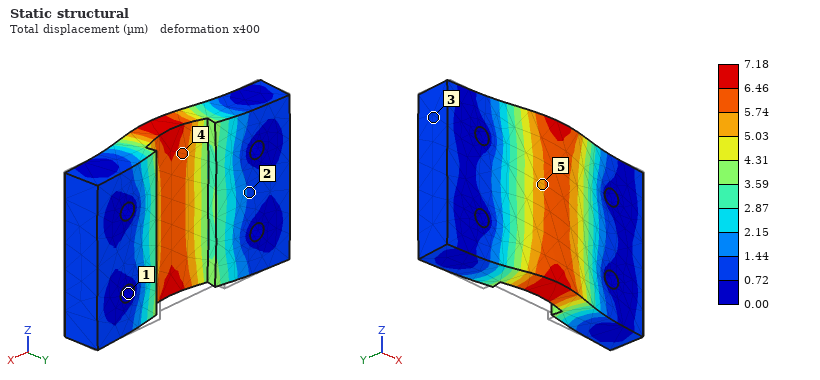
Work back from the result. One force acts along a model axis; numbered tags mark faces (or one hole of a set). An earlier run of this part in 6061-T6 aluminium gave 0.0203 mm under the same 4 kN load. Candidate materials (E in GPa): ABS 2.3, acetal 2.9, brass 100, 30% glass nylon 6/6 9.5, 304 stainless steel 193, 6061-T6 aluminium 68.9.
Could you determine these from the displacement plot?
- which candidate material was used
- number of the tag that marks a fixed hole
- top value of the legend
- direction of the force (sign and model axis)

304 stainless steel
1
7.18 µm
-Y
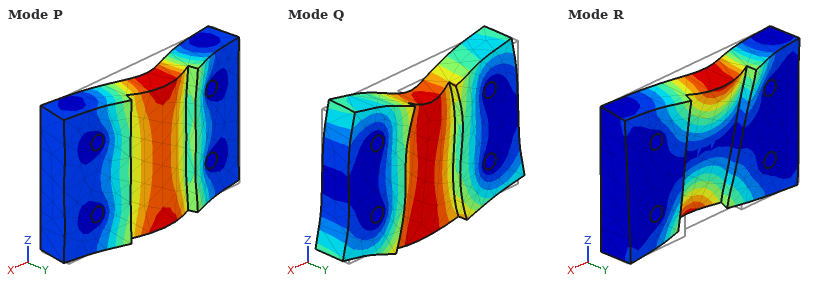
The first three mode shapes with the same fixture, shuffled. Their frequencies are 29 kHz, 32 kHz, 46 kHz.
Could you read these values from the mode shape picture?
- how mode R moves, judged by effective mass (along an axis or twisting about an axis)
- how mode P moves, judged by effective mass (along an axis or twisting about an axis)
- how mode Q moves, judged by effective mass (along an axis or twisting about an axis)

twisting about X
along Y
along Z
